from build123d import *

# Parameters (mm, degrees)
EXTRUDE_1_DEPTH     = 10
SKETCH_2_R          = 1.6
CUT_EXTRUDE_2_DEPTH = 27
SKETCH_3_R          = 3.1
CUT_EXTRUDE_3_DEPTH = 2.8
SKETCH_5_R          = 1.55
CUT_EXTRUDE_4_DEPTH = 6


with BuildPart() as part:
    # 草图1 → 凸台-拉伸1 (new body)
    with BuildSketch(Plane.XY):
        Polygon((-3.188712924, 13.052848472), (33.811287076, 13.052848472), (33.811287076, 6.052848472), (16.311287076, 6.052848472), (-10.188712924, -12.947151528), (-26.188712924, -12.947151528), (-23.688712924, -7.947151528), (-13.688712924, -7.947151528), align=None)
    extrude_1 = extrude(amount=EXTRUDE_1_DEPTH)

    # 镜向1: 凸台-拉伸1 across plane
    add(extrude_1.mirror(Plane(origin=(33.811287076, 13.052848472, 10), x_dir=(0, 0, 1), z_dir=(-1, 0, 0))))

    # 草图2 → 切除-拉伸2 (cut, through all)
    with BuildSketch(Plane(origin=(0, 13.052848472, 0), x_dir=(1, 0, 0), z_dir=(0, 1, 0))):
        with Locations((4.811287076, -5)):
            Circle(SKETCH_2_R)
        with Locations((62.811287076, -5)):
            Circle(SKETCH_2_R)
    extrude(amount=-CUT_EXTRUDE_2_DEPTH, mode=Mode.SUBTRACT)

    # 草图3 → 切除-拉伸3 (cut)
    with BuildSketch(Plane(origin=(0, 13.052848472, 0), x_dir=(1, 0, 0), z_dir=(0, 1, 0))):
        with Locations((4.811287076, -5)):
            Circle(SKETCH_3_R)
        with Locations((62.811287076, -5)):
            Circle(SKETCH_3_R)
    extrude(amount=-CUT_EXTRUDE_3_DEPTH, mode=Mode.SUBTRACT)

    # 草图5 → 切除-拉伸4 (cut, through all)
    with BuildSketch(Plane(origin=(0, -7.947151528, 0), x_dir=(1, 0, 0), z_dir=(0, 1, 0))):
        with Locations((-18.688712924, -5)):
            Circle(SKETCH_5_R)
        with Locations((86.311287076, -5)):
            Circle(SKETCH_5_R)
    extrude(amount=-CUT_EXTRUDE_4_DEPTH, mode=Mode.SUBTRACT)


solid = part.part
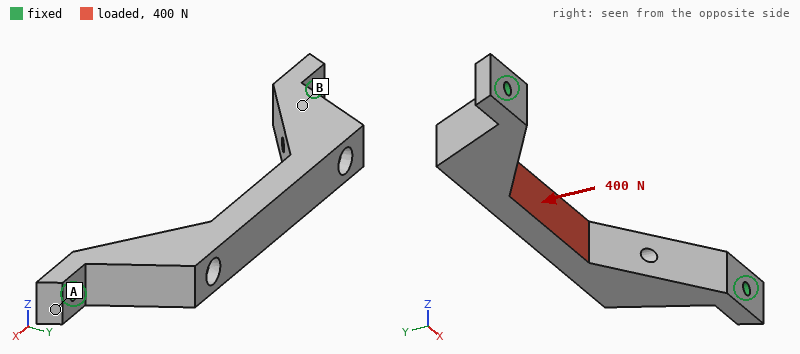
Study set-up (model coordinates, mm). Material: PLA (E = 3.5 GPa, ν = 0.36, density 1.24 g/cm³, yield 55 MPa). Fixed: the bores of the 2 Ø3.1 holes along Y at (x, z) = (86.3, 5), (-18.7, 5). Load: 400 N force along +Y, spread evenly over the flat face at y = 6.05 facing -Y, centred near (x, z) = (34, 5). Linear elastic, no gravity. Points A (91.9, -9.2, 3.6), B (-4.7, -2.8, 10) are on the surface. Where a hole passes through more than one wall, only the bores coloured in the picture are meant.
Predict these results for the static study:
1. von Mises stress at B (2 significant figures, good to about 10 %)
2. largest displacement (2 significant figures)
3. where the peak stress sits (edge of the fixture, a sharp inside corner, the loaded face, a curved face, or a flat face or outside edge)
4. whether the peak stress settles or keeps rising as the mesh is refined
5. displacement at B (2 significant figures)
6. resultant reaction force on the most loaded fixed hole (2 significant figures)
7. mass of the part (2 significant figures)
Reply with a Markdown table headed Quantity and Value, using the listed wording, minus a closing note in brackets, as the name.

| Quantity | Value |
|---|---|
| von Mises stress at B | 4.7 MPa |
| largest displacement | 0.35 mm |
| where the peak stress sits | edge of the fixture |
| whether the peak stress settles or keeps rising as the mesh is refined | keeps rising |
| displacement at B | 0.057 mm |
| resultant reaction force on the most loaded fixed hole | 400 N |
| mass of the part | 14 g |
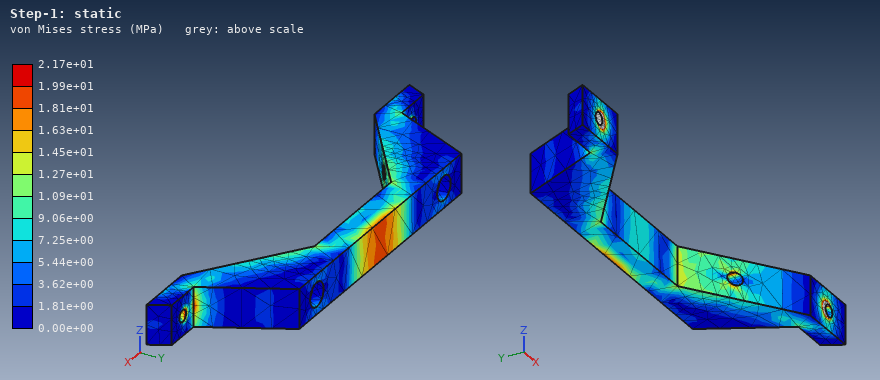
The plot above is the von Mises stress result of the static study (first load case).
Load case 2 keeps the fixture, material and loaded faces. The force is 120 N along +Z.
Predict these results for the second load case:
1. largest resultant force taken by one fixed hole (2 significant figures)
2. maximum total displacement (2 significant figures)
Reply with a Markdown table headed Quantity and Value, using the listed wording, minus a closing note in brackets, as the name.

| Quantity | Value |
|---|---|
| largest resultant force taken by one fixed hole | 60 N |
| maximum total displacement | 0.88 mm |
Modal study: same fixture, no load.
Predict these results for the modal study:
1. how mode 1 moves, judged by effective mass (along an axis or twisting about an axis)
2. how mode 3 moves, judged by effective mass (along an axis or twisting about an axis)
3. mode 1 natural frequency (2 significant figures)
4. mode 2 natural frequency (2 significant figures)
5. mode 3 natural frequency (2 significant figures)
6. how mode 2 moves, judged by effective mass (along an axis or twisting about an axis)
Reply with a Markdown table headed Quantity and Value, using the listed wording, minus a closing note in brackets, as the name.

| Quantity | Value |
|---|---|
| how mode 1 moves, judged by effective mass | along Z |
| how mode 3 moves, judged by effective mass | along X |
| mode 1 natural frequency | 720 Hz |
| mode 2 natural frequency | 1800 Hz |
| mode 3 natural frequency | 1900 Hz |
| how mode 2 moves, judged by effective mass | twisting about Y |
